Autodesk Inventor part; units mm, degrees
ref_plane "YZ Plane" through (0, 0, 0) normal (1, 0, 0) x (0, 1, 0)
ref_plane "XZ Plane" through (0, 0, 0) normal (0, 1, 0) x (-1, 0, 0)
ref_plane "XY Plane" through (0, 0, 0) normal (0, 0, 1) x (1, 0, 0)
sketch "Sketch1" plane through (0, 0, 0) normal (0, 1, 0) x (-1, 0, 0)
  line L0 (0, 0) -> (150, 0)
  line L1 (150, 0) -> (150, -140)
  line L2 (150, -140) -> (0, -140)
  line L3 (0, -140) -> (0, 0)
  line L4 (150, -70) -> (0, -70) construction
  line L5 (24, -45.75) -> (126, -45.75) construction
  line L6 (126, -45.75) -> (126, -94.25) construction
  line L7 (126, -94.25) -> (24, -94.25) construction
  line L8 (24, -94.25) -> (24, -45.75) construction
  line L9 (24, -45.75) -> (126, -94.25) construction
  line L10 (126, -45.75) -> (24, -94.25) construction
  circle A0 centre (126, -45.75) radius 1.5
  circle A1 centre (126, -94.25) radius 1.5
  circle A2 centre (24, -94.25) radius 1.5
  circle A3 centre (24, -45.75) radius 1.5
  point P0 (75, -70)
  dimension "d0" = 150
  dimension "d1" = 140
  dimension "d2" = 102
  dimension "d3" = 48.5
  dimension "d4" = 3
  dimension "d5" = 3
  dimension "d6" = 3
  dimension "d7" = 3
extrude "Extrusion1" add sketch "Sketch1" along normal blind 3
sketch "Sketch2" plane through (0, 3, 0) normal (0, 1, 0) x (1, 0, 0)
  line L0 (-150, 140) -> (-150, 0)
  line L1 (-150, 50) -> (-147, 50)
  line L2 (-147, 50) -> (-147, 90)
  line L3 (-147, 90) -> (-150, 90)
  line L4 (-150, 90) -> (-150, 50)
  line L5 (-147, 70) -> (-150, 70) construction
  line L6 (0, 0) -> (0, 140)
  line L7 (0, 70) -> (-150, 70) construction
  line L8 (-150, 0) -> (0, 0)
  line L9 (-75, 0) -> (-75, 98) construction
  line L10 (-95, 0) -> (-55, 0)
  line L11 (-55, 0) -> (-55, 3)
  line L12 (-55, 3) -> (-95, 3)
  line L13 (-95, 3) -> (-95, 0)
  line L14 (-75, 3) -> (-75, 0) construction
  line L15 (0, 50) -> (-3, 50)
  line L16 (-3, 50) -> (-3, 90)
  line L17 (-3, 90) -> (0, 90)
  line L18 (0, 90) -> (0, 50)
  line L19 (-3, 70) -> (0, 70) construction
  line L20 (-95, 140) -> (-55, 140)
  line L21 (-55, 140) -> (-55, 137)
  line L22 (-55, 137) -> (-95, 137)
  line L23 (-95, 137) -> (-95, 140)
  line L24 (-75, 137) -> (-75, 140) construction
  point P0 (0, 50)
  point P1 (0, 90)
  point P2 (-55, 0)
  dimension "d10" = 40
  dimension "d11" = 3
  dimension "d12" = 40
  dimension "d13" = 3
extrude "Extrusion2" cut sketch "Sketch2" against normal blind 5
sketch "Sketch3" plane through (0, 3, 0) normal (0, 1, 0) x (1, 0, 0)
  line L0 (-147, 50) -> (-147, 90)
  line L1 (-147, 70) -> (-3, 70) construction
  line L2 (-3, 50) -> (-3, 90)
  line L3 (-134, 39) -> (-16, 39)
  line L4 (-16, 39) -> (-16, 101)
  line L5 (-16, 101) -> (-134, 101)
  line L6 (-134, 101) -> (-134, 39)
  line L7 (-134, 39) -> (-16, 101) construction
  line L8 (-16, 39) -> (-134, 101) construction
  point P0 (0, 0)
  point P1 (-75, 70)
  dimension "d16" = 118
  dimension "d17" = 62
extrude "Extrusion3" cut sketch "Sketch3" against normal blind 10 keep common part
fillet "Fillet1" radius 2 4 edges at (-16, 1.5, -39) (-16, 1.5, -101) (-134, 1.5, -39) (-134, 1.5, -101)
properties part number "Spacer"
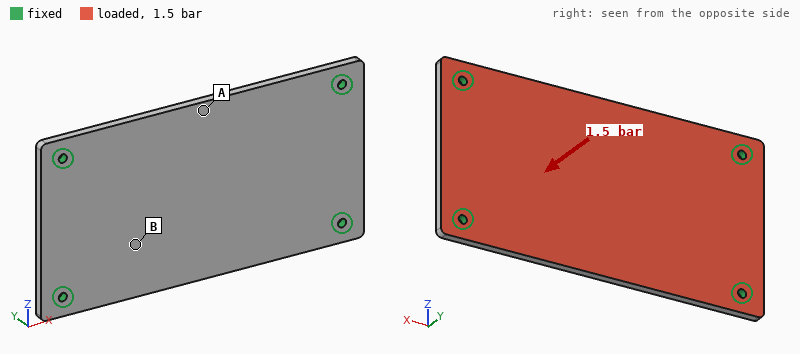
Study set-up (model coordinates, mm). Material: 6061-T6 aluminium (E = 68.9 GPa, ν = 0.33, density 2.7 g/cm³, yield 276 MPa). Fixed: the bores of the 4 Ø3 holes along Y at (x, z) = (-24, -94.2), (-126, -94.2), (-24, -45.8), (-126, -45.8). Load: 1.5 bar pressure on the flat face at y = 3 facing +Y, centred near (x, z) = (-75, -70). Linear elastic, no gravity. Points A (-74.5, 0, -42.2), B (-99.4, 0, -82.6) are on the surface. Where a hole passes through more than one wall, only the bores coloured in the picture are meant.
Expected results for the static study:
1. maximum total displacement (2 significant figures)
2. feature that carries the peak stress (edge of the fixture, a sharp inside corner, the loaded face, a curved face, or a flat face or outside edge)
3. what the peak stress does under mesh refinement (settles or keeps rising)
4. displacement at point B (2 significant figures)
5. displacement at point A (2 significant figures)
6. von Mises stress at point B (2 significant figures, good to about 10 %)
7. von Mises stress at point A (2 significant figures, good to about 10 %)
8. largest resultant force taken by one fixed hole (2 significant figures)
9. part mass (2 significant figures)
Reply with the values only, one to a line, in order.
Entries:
0.36 mm
edge of the fixture
keeps rising
0.23 mm
0.35 mm
21 MPa
52 MPa
270 N
59 g
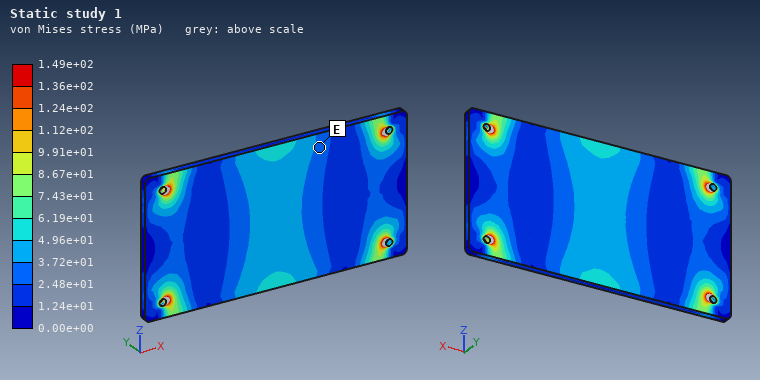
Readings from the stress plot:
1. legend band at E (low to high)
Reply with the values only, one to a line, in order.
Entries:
2.48e+01 to 3.72e+01 MPa
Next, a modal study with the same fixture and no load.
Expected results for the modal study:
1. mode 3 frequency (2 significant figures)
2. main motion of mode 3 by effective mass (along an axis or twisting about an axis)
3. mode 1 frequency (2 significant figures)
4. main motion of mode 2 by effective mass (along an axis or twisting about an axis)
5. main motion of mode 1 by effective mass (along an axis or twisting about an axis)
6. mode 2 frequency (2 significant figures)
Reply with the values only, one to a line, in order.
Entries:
3600 Hz
twisting about Z
1300 Hz
twisting about X
along Y
2200 Hz
